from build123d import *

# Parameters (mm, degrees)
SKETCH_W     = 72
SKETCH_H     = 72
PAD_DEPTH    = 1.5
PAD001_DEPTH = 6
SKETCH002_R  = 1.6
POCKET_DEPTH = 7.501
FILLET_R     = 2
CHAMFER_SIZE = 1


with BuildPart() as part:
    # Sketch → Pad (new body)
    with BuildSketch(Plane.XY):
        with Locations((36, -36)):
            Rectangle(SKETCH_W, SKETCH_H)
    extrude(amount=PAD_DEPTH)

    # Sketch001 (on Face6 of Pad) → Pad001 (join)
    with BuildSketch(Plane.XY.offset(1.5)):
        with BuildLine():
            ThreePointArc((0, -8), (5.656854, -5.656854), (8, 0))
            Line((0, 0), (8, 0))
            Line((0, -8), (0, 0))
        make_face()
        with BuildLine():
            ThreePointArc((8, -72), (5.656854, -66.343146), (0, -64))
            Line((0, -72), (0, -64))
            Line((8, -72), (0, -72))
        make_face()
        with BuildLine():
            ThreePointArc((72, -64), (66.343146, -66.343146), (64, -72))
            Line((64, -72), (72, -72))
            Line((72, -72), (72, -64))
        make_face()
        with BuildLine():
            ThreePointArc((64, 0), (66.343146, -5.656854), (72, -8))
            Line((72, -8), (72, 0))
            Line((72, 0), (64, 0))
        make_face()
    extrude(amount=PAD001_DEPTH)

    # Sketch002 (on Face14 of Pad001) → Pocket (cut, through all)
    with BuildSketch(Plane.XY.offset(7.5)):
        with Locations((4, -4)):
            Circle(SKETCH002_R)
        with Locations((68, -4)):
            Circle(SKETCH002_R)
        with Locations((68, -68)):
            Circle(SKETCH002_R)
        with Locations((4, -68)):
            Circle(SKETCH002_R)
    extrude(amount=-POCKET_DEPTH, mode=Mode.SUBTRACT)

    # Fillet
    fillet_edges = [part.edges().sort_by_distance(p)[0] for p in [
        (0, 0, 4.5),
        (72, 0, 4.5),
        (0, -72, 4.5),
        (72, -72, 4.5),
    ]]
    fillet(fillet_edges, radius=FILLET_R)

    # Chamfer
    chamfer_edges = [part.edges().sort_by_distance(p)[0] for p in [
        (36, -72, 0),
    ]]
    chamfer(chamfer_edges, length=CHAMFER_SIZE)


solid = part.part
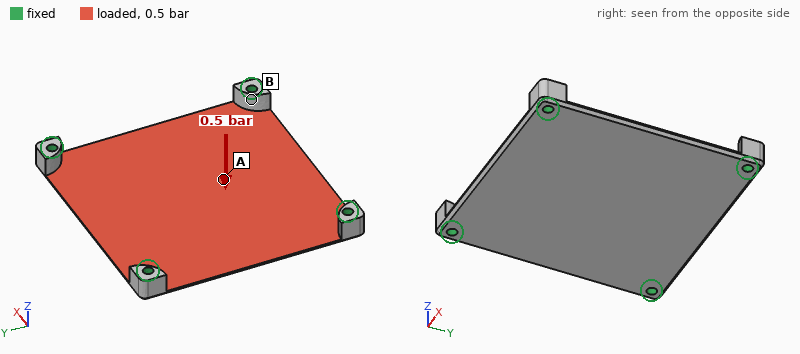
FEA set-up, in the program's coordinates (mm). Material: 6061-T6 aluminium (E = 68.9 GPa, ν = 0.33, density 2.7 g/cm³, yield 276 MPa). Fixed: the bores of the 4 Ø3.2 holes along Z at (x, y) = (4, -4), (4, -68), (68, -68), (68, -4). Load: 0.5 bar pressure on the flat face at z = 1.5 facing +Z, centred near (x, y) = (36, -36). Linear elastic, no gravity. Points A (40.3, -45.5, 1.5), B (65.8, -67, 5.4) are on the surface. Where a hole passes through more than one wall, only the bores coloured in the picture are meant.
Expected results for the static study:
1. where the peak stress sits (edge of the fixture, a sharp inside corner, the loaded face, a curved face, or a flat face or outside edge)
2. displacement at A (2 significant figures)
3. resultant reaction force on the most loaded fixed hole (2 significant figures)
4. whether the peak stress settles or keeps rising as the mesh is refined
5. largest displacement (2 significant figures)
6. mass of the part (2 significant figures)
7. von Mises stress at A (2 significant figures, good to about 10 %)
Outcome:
edge of the fixture
0.26 mm
70 N
keeps rising
0.28 mm
23 g
27 MPa
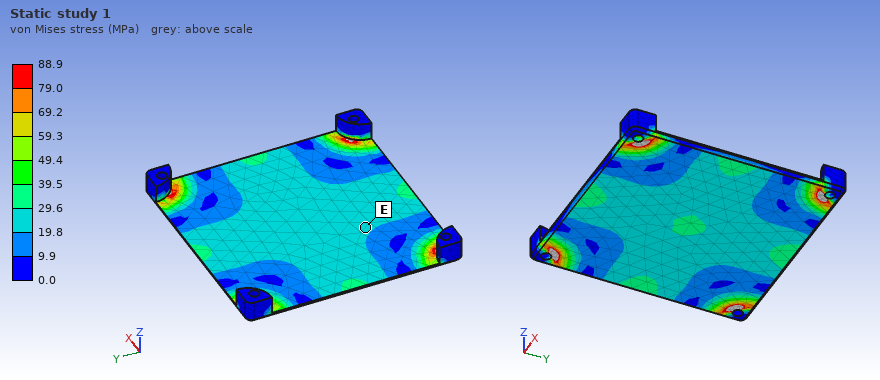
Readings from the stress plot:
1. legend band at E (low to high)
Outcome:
19.8 to 29.6 MPa
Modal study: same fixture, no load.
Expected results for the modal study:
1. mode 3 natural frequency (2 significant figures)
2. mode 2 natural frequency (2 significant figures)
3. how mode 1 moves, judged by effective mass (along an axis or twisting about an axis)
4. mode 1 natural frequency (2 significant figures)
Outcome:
2300 Hz
2300 Hz
along Z
1300 Hz
